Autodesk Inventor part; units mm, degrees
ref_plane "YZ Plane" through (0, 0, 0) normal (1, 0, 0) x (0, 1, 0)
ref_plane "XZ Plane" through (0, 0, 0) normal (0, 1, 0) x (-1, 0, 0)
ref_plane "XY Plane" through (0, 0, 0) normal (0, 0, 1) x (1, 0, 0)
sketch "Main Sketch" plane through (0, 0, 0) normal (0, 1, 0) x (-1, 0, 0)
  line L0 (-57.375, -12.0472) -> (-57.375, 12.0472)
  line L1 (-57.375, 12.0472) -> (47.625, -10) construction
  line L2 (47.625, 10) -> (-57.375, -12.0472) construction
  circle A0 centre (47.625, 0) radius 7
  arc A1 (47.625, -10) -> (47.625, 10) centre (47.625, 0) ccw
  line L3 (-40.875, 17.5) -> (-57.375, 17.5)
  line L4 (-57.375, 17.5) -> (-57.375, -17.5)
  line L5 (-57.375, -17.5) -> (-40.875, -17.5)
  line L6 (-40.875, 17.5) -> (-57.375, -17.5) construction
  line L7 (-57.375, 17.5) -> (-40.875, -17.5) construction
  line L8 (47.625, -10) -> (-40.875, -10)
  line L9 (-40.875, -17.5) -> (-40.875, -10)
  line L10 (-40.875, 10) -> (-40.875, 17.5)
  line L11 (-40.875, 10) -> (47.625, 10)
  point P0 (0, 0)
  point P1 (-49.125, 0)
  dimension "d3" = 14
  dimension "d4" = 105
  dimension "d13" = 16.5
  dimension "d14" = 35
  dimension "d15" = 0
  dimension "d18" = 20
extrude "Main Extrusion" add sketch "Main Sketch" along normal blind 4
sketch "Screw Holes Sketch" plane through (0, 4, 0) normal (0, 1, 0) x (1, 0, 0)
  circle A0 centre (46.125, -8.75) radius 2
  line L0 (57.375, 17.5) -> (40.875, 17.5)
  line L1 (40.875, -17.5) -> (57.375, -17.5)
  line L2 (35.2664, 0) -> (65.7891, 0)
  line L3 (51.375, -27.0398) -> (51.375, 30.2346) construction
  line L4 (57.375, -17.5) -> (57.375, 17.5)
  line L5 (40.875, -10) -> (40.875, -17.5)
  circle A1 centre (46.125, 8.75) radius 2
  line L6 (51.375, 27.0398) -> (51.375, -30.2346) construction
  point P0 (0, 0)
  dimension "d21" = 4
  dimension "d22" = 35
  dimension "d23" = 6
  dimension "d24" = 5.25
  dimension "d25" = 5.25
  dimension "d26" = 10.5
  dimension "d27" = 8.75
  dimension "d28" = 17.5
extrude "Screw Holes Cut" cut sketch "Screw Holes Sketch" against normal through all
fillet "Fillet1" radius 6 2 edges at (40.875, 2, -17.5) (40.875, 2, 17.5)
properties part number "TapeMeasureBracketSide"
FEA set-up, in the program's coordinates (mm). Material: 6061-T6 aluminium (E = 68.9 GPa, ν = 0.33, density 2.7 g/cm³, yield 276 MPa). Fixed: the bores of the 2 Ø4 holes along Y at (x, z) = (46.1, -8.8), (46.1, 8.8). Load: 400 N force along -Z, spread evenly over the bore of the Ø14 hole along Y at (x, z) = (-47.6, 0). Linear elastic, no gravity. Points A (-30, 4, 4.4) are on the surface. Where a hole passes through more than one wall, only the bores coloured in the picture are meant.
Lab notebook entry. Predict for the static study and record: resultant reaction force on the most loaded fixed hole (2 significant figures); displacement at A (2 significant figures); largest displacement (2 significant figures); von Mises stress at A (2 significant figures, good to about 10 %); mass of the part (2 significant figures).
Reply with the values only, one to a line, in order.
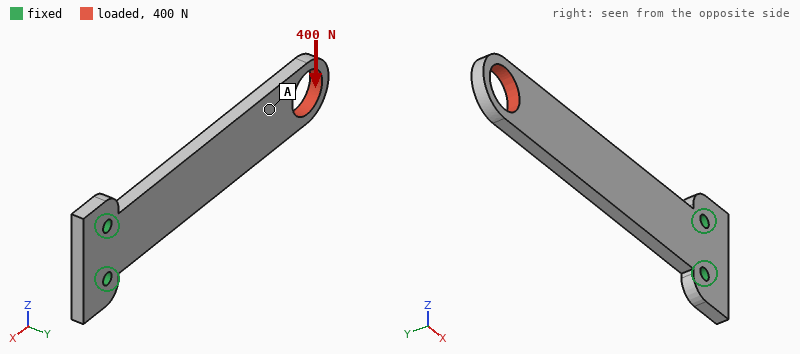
2.1 kN
0.42 mm
0.69 mm
15 MPa
25 g
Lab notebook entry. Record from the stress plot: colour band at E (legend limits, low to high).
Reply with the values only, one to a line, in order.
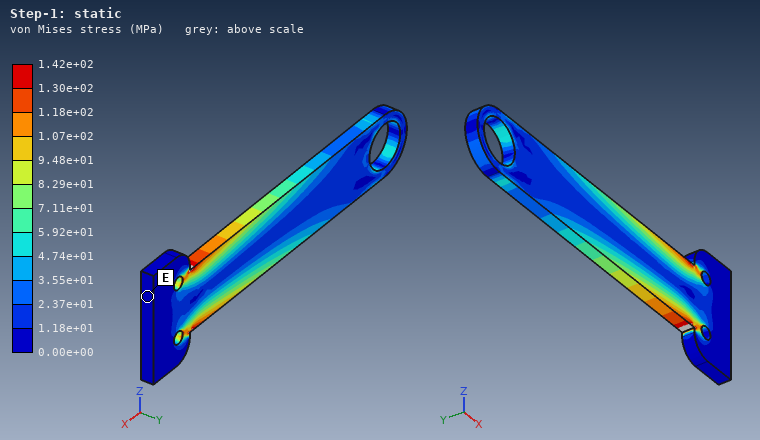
0.00e+00 to 1.18e+01 MPa
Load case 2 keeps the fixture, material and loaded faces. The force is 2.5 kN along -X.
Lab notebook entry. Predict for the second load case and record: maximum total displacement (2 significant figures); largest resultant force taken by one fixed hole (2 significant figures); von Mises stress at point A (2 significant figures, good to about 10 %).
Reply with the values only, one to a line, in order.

77 µm
1.3 kN
29 MPa
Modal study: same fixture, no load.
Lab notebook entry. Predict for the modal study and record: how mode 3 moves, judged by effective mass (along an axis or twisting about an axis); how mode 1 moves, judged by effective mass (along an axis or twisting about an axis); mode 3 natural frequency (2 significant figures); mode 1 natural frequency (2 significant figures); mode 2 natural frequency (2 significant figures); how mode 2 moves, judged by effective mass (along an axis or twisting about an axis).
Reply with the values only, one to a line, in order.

along Y
along Y
2200 Hz
370 Hz
1800 Hz
along Z
